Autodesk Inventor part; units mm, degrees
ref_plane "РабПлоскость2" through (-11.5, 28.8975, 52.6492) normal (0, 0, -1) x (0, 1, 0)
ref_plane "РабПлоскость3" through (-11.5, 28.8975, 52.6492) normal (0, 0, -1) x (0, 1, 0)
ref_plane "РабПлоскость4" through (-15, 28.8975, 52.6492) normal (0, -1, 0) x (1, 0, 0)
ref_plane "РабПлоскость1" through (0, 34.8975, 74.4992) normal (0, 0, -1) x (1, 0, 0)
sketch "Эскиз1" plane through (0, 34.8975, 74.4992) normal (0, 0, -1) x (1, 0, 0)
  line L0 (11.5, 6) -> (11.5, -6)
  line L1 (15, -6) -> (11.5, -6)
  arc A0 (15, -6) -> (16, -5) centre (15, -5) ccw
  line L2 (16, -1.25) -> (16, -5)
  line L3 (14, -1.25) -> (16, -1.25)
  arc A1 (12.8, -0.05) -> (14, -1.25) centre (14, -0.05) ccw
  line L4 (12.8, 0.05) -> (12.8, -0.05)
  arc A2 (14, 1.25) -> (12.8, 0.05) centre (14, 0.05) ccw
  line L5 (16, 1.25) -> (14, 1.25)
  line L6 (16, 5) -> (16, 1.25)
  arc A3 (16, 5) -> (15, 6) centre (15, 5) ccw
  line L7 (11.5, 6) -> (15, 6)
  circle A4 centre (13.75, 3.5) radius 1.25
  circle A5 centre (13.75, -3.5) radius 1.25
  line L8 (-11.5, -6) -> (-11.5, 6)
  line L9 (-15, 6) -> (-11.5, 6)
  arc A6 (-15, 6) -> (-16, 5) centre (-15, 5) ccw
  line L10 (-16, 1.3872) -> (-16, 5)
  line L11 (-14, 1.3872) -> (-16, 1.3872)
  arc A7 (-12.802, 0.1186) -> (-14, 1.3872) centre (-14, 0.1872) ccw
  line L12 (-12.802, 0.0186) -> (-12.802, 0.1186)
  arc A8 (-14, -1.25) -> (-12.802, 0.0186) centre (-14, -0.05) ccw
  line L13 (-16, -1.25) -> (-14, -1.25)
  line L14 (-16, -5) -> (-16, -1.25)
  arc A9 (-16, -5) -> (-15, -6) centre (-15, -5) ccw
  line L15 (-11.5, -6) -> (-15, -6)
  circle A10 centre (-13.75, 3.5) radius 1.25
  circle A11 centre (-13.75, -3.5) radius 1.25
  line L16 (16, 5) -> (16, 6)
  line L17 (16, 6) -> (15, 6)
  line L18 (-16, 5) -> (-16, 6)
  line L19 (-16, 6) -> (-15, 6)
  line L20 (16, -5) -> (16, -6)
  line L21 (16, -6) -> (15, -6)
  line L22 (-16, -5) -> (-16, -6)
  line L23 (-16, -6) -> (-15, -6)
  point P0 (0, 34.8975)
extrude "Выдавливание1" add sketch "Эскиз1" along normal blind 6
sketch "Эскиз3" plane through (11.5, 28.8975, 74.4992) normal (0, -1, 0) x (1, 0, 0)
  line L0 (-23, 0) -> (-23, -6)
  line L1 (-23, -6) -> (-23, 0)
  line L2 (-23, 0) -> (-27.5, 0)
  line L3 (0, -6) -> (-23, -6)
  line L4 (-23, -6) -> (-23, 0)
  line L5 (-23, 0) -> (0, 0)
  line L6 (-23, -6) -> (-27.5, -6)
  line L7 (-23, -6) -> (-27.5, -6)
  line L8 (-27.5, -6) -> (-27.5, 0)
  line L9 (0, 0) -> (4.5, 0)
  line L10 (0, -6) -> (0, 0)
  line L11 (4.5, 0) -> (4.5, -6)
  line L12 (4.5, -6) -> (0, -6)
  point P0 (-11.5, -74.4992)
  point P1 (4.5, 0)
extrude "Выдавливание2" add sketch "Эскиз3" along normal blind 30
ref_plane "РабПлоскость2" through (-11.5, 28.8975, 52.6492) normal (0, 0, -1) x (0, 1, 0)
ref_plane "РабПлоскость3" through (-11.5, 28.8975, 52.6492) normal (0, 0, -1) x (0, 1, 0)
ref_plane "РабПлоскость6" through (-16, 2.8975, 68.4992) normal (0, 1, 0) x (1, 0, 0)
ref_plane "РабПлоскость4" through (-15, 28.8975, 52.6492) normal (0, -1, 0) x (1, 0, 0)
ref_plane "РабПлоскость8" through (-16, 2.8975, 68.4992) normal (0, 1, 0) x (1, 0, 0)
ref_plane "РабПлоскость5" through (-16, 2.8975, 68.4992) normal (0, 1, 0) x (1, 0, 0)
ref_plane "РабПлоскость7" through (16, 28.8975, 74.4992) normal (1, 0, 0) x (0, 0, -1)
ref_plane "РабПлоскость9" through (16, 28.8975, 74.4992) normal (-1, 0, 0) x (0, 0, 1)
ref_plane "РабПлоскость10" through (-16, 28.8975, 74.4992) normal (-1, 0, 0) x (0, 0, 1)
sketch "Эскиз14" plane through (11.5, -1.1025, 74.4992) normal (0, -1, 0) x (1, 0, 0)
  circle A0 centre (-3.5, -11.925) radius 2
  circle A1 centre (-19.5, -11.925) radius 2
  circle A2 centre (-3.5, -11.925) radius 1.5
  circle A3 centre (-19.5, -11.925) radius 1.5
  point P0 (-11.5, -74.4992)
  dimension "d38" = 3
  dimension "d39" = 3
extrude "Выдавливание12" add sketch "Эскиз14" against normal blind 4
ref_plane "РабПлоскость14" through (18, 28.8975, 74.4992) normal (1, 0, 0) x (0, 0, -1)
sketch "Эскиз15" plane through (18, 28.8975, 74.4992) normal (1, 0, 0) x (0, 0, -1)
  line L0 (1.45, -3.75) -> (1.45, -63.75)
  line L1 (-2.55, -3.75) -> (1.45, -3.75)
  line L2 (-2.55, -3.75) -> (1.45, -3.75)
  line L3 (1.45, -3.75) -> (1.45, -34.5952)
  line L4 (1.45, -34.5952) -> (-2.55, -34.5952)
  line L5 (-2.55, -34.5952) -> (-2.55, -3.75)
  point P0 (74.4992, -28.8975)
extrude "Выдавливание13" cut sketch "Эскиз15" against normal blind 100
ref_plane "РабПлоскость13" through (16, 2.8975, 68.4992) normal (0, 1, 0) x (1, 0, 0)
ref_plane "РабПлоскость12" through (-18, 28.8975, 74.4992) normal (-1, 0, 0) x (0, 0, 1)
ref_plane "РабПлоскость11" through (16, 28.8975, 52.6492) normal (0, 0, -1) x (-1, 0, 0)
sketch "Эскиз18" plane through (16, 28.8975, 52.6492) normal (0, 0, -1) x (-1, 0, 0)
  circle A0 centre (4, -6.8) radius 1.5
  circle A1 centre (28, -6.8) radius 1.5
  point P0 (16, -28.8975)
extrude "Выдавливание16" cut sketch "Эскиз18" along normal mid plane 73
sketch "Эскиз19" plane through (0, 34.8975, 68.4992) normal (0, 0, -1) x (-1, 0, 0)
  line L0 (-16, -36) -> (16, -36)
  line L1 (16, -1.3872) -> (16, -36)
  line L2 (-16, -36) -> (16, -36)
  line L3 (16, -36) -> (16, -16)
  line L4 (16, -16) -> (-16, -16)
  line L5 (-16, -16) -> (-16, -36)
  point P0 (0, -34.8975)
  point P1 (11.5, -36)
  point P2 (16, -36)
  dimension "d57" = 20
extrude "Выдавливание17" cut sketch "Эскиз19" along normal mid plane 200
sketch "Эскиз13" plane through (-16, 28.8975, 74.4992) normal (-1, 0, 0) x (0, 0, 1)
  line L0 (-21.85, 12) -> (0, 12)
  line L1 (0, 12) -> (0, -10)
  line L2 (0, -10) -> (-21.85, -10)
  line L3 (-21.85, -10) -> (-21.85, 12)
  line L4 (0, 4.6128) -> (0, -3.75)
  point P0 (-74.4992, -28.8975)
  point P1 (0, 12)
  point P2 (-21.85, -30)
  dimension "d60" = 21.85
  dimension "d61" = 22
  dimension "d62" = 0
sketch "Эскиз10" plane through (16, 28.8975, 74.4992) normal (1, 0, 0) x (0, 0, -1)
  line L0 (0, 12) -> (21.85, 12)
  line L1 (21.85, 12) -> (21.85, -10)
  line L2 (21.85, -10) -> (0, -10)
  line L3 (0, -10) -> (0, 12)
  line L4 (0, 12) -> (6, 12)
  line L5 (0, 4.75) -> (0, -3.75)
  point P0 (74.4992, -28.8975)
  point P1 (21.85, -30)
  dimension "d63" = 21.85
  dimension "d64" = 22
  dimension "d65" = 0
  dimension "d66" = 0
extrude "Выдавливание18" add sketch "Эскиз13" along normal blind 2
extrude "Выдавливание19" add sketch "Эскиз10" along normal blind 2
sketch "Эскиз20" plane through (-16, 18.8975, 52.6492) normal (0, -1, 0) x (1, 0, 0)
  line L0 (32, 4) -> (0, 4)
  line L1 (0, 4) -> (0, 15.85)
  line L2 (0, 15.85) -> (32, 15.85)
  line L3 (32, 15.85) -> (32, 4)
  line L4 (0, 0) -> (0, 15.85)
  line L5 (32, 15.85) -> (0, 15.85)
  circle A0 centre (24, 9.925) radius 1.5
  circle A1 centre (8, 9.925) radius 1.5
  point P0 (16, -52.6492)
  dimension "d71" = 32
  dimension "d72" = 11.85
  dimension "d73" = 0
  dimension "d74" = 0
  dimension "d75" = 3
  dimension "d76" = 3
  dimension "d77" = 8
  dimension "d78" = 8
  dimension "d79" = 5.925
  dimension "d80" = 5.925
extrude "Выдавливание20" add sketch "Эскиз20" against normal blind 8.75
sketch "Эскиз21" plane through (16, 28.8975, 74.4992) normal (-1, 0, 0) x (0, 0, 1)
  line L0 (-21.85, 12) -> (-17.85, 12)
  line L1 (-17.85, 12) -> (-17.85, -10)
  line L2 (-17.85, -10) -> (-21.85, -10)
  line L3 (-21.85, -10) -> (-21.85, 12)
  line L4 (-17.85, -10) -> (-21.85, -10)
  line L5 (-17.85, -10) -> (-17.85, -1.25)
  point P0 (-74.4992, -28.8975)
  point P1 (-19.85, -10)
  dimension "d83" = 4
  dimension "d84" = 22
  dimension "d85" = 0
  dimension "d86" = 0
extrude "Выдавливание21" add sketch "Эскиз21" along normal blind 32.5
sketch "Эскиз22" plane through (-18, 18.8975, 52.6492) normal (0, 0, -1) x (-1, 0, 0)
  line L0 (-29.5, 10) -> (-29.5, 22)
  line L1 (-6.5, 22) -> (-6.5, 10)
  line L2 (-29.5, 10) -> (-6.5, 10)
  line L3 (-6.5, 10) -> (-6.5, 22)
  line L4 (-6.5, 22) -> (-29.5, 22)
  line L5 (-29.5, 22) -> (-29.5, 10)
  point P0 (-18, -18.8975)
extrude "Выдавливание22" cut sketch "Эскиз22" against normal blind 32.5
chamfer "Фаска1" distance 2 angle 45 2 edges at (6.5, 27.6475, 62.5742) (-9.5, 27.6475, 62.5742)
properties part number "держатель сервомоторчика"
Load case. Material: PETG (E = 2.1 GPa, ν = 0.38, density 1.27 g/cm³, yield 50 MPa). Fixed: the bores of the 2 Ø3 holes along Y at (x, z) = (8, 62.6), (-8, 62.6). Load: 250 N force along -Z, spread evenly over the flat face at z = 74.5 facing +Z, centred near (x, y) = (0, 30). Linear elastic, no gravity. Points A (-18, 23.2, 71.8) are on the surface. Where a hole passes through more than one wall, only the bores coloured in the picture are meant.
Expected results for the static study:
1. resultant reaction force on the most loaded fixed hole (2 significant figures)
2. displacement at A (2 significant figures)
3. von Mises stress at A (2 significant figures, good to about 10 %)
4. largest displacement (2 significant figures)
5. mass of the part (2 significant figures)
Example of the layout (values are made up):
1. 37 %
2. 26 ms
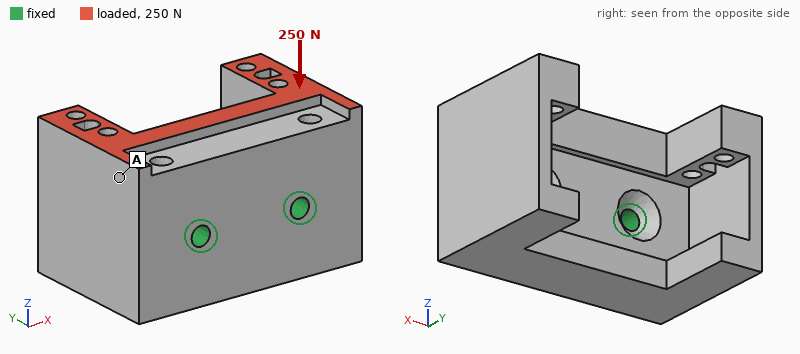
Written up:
1. 130 N
2. 0.045 mm
3. 1.7 MPa
4. 0.16 mm
5. 11 g
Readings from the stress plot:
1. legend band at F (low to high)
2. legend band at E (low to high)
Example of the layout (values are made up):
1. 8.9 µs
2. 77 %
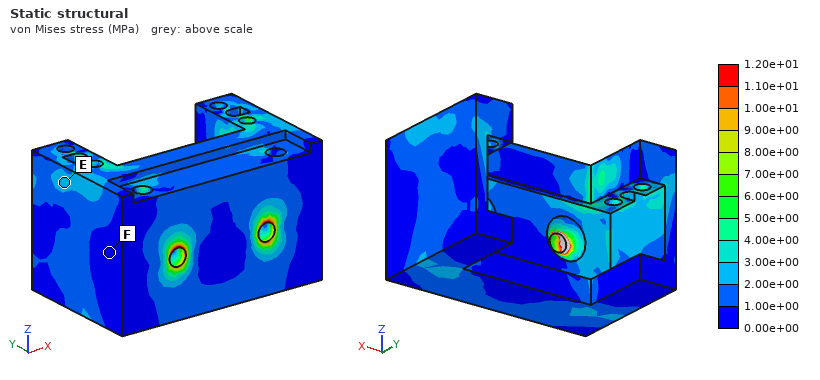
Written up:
1. 0.00e+00 to 1.00e+00 MPa
2. 2.00e+00 to 3.00e+00 MPa
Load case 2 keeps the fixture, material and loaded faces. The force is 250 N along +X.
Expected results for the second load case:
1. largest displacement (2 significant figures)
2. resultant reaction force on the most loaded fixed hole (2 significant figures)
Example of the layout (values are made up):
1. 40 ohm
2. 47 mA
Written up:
1. 0.26 mm
2. 220 N
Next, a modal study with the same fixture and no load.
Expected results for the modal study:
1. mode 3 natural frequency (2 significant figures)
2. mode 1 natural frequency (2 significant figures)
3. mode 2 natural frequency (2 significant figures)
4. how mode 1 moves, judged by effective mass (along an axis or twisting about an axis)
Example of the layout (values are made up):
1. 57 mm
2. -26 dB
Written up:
1. 3700 Hz
2. 3300 Hz
3. 3500 Hz
4. along Z
